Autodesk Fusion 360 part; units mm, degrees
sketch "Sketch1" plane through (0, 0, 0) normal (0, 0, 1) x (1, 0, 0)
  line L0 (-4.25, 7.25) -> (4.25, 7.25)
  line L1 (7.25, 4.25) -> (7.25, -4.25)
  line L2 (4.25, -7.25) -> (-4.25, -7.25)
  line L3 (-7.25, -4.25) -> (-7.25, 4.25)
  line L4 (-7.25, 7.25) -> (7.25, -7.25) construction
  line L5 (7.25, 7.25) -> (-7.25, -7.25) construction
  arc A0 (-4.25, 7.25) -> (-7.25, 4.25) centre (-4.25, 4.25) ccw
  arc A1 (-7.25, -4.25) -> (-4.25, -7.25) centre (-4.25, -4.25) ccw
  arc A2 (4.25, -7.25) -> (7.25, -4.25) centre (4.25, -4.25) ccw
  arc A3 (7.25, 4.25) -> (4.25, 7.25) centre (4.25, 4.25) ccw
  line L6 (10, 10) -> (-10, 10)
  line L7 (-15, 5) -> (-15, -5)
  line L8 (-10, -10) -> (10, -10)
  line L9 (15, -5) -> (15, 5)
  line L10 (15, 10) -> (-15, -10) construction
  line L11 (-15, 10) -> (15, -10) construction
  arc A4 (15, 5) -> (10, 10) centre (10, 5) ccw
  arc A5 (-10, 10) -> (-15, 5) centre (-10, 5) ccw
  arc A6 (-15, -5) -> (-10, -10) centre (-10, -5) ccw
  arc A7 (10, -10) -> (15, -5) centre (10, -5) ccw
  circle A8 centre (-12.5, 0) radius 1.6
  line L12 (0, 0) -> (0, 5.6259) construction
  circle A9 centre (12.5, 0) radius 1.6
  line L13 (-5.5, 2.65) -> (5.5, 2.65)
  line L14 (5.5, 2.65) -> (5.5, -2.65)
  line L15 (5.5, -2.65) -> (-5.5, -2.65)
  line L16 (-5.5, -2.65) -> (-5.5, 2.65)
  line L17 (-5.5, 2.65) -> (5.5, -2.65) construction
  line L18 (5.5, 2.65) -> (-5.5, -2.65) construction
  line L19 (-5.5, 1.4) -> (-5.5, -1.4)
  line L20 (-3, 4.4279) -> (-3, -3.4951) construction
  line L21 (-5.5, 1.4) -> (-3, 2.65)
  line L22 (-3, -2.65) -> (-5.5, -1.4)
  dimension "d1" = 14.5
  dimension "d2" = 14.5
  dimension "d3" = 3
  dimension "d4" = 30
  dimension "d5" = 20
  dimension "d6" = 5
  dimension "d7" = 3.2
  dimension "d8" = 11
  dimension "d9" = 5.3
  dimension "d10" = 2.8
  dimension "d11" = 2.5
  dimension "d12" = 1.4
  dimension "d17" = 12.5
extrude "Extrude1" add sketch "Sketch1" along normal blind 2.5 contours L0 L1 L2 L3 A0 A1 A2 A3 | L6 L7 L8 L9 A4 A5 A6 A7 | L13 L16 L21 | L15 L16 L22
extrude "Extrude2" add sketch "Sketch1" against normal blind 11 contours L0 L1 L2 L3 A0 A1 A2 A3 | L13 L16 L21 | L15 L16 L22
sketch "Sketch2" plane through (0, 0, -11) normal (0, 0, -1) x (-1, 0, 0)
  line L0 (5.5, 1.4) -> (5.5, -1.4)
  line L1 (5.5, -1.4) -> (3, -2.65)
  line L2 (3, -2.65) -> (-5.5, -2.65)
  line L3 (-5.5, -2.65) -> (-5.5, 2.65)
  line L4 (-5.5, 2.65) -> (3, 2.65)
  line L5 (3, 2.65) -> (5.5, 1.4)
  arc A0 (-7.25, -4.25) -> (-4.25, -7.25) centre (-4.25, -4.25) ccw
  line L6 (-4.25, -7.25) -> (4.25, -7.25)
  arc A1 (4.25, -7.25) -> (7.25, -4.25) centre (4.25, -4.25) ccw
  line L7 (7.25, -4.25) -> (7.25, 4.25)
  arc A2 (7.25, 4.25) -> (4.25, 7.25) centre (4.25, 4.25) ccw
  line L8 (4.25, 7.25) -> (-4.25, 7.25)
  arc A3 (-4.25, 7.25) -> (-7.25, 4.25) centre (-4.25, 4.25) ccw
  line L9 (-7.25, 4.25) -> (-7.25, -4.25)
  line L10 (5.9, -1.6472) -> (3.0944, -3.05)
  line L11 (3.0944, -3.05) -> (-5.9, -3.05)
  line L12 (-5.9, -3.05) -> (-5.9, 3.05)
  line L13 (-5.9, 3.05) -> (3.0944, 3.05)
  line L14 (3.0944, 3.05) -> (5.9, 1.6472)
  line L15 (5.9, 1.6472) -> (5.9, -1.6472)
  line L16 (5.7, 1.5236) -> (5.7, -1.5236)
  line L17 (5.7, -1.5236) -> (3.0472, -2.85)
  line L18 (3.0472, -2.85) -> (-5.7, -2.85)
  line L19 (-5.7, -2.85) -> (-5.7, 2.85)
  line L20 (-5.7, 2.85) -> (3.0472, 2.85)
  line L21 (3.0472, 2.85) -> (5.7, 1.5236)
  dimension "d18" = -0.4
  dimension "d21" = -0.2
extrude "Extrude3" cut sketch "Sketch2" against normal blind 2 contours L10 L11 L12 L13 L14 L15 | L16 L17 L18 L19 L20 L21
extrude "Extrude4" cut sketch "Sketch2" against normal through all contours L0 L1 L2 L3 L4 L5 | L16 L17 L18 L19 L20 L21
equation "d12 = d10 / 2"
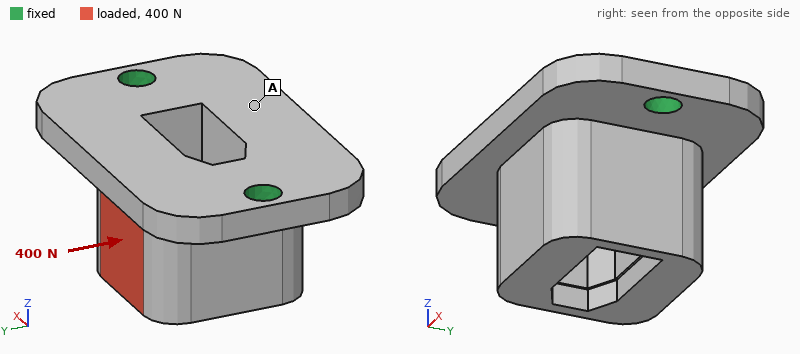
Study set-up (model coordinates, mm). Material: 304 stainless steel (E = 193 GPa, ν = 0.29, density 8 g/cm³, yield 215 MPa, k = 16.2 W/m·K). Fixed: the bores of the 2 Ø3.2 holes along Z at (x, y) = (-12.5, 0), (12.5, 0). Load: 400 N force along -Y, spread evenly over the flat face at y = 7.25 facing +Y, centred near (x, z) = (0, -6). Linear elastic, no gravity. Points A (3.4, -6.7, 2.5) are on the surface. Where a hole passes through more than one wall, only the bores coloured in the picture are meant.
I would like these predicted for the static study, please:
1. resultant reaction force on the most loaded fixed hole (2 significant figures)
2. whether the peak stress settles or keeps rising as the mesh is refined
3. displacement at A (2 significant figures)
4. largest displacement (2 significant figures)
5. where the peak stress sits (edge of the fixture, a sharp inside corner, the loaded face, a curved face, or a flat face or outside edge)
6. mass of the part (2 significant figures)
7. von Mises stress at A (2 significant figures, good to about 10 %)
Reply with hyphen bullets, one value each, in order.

- 200 N
- keeps rising
- 7.2 µm
- 18 µm
- edge of the fixture
- 22 g
- 16 MPa
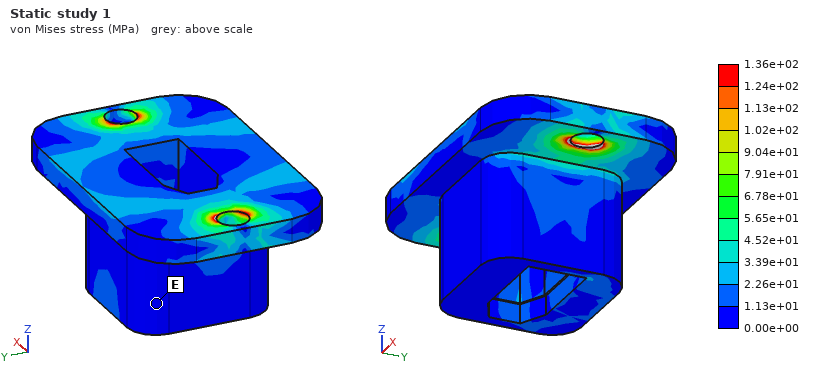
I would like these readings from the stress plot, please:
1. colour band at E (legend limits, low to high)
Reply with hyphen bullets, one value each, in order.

- 0.00e+00 to 1.13e+01 MPa
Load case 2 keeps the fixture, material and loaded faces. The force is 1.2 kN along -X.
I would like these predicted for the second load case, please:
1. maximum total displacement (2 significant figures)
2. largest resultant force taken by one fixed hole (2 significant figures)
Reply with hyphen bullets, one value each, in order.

- 9.6 µm
- 810 N
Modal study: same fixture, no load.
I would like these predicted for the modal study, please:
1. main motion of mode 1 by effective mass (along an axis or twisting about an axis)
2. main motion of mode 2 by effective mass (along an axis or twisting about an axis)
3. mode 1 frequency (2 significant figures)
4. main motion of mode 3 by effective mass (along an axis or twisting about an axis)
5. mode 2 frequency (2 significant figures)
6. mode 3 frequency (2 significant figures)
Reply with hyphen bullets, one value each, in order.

- along Y
- along Z
- 7000 Hz
- along X
- 16 kHz
- 19 kHz
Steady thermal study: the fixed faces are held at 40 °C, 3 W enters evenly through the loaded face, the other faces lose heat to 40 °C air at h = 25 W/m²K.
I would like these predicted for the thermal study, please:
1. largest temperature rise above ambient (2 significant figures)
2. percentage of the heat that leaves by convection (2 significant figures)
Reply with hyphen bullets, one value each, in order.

- 35 K
- 24 %
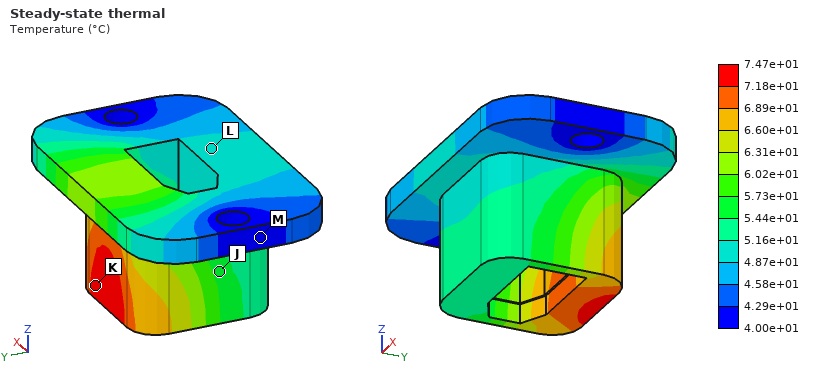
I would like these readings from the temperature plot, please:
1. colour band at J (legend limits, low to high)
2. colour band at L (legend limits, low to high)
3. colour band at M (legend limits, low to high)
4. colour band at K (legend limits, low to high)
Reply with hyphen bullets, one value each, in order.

- 5.44e+01 to 5.73e+01 °C
- 4.87e+01 to 5.16e+01 °C
- 4.00e+01 to 4.29e+01 °C
- 7.18e+01 to 7.47e+01 °C
